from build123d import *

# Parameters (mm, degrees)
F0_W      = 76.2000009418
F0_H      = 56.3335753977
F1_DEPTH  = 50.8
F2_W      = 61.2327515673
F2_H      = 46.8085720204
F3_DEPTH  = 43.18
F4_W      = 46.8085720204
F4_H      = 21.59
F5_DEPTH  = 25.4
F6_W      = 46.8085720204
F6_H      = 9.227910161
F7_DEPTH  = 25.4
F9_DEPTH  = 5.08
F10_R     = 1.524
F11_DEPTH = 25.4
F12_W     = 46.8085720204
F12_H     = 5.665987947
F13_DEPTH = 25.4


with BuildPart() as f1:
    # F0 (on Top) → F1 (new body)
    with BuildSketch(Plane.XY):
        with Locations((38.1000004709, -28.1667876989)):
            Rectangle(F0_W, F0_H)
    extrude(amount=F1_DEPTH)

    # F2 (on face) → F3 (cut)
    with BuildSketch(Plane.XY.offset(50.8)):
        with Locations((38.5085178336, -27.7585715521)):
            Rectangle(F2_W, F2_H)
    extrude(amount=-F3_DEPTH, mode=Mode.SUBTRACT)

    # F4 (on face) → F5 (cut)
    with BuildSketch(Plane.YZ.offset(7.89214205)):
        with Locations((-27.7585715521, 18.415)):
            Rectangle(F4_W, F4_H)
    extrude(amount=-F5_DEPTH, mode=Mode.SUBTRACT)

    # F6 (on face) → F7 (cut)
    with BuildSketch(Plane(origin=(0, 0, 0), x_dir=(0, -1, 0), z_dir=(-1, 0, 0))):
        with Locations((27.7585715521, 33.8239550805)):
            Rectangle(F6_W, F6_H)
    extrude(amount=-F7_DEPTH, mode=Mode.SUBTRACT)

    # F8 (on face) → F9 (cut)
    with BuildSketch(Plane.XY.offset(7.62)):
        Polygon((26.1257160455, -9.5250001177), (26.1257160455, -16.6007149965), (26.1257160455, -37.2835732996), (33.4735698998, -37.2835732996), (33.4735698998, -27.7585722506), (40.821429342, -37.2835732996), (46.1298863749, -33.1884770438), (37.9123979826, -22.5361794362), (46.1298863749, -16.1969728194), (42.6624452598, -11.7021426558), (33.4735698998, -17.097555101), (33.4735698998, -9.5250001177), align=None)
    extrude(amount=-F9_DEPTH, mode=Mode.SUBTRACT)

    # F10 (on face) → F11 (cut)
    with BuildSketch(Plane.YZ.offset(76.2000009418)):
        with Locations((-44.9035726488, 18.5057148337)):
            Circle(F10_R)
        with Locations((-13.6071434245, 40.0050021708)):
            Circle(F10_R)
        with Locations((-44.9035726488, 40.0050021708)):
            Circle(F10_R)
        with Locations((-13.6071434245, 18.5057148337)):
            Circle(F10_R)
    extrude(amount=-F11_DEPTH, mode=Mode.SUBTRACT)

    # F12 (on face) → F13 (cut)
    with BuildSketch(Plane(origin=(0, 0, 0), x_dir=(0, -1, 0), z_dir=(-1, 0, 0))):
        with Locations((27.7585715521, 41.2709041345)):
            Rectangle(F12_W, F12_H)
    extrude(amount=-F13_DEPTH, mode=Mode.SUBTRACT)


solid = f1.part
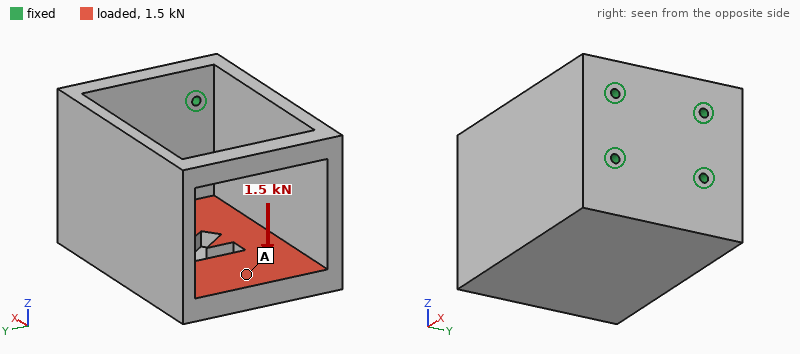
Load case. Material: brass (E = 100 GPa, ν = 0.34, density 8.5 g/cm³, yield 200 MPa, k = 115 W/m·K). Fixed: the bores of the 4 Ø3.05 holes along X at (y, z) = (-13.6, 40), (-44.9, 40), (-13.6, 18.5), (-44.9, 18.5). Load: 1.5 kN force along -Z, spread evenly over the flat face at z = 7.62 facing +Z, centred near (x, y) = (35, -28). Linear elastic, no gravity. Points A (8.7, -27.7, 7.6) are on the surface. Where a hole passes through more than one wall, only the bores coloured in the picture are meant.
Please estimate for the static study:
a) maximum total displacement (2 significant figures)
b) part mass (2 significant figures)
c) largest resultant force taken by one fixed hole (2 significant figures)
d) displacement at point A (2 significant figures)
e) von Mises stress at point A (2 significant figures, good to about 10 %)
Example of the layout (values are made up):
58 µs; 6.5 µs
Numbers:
55 µm; 670 g; 1.2 kN; 47 µm; 11 MPa
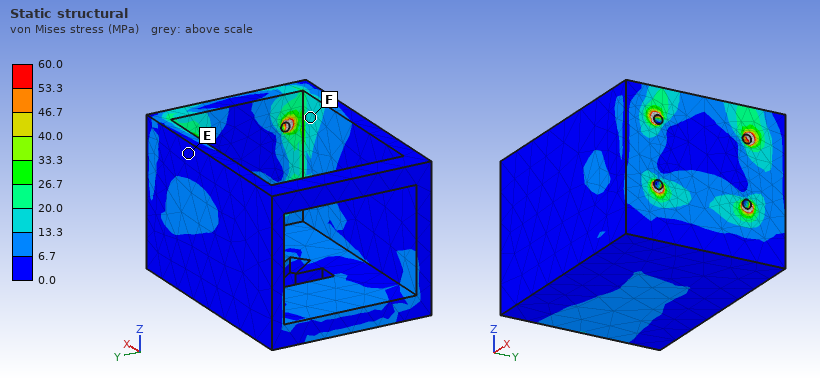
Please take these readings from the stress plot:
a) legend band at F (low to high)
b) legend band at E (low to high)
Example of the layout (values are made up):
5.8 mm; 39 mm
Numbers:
13.3 to 20.0 MPa; 0.0 to 6.7 MPa
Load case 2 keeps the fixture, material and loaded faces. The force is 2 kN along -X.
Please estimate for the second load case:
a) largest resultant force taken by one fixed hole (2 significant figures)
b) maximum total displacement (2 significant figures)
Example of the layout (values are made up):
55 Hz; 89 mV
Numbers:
1.3 kN; 26 µm
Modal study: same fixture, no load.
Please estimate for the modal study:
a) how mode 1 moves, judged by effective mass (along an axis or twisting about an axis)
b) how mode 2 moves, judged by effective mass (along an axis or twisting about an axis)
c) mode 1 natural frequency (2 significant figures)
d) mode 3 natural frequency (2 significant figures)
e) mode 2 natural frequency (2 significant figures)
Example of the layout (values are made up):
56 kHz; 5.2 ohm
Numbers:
along Y; along Z; 1000 Hz; 2500 Hz; 1500 Hz
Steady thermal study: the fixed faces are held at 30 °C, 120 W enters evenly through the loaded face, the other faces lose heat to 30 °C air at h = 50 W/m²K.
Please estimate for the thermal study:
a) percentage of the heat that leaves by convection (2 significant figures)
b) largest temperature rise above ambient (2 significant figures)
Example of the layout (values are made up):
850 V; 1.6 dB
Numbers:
31 %; 61 K
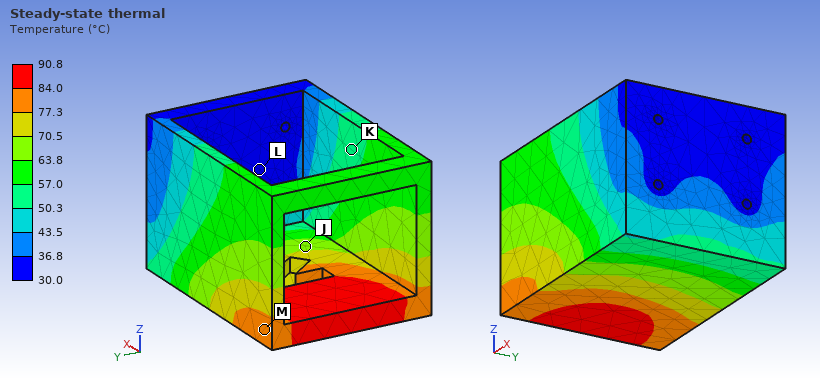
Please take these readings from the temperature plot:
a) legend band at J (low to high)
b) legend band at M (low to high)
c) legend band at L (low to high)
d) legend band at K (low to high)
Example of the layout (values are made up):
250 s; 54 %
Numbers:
63.8 to 70.5 °C; 77.3 to 84.0 °C; 30.0 to 36.8 °C; 50.3 to 57.0 °C
